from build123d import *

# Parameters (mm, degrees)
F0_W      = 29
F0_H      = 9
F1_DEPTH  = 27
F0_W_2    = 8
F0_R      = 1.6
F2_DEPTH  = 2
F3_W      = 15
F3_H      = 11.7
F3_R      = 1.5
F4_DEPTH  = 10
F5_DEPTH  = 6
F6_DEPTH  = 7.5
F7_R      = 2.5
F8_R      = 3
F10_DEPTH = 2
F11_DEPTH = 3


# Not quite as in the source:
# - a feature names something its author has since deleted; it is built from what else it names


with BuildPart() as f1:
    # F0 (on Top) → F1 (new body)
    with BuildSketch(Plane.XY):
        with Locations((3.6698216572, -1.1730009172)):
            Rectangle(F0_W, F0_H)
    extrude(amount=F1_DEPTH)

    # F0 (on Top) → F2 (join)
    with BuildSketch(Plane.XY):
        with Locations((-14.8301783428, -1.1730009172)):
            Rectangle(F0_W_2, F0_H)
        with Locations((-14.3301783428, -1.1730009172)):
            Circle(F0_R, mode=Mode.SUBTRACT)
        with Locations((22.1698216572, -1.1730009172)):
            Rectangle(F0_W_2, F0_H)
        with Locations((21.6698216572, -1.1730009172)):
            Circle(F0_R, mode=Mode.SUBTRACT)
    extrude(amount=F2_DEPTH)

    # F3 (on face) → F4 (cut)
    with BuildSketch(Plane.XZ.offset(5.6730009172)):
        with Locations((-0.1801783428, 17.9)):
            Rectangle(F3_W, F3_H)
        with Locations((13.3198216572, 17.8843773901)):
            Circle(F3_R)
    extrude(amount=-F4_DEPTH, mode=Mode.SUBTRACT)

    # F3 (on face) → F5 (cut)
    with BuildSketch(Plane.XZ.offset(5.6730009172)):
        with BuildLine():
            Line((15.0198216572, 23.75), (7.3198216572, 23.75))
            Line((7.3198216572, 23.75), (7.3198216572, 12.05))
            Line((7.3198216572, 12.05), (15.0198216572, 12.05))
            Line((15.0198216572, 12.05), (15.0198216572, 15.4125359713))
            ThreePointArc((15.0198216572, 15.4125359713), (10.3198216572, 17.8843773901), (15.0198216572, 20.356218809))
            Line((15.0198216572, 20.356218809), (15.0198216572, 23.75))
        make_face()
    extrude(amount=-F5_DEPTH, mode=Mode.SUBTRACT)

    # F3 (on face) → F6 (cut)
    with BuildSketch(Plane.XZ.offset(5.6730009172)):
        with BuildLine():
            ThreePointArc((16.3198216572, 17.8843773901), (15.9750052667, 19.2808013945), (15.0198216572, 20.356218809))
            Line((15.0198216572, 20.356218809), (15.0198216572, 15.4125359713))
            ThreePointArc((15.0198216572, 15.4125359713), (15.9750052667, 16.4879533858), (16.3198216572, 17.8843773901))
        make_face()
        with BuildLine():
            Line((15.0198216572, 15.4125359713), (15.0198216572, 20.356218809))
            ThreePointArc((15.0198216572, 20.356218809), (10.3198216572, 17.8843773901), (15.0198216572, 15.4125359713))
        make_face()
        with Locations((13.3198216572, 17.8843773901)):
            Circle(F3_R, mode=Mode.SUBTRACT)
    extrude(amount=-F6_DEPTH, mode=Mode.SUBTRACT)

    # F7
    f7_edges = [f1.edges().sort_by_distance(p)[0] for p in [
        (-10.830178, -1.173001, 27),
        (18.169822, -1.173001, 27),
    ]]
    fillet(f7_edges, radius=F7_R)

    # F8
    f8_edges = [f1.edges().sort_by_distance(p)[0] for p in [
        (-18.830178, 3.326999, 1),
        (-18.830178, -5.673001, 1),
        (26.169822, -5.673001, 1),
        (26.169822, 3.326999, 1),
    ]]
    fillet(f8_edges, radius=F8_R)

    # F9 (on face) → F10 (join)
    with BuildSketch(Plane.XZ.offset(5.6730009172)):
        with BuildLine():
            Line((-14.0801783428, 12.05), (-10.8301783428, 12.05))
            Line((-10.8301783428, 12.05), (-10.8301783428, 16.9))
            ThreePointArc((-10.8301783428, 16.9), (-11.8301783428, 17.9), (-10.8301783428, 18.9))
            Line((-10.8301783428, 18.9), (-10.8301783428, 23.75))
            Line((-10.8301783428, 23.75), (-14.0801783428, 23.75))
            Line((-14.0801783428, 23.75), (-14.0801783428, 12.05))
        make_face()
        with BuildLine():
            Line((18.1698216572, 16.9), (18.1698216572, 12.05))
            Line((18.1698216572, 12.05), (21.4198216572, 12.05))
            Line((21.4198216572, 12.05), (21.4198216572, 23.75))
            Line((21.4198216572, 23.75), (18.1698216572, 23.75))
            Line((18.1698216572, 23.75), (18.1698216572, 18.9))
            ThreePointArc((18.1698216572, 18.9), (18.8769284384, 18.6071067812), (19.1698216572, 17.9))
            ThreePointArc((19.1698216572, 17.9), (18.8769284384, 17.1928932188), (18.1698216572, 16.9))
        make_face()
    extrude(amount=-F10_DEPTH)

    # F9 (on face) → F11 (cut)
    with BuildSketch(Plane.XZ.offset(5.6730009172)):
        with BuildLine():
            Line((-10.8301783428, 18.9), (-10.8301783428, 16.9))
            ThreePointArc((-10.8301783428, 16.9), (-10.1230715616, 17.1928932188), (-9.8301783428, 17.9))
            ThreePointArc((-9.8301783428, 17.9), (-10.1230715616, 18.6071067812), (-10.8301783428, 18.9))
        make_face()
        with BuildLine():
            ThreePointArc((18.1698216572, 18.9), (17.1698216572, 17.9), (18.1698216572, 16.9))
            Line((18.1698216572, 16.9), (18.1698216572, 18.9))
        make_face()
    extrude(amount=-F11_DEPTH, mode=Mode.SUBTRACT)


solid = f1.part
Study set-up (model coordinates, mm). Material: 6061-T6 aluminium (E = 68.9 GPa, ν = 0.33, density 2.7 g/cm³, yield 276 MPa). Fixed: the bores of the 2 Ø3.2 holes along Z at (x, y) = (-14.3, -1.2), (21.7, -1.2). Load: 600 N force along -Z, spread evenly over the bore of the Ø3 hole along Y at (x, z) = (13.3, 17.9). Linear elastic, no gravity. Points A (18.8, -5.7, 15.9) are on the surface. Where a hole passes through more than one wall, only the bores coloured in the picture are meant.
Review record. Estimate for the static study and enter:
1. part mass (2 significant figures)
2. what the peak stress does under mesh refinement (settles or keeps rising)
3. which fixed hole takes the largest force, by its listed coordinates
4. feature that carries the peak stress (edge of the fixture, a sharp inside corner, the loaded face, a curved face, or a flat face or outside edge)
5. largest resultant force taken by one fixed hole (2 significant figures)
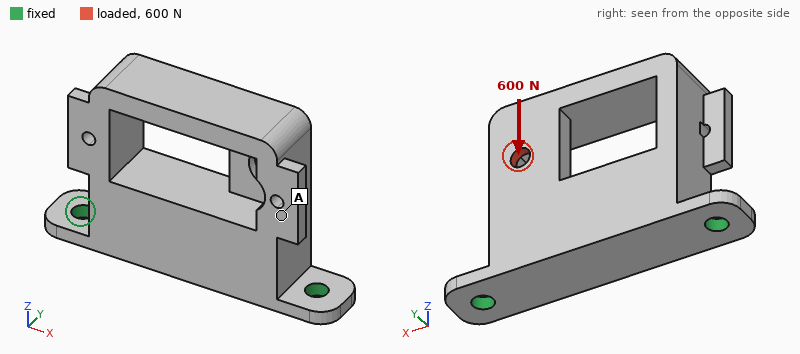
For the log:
14 g
keeps rising
(21.7, -1.2)
edge of the fixture
520 N
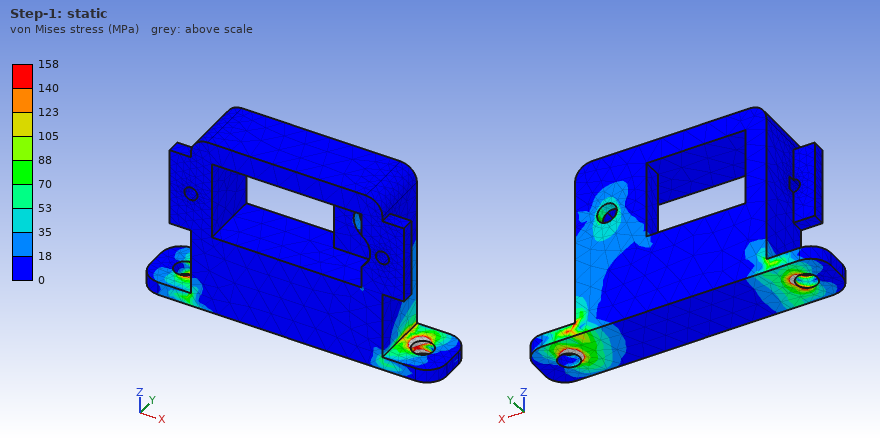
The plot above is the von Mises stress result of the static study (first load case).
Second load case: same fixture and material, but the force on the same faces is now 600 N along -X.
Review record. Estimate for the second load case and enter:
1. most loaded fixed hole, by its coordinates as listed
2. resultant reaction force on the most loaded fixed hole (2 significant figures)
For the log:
(-14.3, -1.2)
500 N
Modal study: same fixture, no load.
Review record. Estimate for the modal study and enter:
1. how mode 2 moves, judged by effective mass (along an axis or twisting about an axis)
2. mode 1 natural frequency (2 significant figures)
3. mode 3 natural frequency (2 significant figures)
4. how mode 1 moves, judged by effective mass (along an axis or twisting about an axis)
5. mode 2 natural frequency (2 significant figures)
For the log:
along X
2200 Hz
11 kHz
along Y
8600 Hz
